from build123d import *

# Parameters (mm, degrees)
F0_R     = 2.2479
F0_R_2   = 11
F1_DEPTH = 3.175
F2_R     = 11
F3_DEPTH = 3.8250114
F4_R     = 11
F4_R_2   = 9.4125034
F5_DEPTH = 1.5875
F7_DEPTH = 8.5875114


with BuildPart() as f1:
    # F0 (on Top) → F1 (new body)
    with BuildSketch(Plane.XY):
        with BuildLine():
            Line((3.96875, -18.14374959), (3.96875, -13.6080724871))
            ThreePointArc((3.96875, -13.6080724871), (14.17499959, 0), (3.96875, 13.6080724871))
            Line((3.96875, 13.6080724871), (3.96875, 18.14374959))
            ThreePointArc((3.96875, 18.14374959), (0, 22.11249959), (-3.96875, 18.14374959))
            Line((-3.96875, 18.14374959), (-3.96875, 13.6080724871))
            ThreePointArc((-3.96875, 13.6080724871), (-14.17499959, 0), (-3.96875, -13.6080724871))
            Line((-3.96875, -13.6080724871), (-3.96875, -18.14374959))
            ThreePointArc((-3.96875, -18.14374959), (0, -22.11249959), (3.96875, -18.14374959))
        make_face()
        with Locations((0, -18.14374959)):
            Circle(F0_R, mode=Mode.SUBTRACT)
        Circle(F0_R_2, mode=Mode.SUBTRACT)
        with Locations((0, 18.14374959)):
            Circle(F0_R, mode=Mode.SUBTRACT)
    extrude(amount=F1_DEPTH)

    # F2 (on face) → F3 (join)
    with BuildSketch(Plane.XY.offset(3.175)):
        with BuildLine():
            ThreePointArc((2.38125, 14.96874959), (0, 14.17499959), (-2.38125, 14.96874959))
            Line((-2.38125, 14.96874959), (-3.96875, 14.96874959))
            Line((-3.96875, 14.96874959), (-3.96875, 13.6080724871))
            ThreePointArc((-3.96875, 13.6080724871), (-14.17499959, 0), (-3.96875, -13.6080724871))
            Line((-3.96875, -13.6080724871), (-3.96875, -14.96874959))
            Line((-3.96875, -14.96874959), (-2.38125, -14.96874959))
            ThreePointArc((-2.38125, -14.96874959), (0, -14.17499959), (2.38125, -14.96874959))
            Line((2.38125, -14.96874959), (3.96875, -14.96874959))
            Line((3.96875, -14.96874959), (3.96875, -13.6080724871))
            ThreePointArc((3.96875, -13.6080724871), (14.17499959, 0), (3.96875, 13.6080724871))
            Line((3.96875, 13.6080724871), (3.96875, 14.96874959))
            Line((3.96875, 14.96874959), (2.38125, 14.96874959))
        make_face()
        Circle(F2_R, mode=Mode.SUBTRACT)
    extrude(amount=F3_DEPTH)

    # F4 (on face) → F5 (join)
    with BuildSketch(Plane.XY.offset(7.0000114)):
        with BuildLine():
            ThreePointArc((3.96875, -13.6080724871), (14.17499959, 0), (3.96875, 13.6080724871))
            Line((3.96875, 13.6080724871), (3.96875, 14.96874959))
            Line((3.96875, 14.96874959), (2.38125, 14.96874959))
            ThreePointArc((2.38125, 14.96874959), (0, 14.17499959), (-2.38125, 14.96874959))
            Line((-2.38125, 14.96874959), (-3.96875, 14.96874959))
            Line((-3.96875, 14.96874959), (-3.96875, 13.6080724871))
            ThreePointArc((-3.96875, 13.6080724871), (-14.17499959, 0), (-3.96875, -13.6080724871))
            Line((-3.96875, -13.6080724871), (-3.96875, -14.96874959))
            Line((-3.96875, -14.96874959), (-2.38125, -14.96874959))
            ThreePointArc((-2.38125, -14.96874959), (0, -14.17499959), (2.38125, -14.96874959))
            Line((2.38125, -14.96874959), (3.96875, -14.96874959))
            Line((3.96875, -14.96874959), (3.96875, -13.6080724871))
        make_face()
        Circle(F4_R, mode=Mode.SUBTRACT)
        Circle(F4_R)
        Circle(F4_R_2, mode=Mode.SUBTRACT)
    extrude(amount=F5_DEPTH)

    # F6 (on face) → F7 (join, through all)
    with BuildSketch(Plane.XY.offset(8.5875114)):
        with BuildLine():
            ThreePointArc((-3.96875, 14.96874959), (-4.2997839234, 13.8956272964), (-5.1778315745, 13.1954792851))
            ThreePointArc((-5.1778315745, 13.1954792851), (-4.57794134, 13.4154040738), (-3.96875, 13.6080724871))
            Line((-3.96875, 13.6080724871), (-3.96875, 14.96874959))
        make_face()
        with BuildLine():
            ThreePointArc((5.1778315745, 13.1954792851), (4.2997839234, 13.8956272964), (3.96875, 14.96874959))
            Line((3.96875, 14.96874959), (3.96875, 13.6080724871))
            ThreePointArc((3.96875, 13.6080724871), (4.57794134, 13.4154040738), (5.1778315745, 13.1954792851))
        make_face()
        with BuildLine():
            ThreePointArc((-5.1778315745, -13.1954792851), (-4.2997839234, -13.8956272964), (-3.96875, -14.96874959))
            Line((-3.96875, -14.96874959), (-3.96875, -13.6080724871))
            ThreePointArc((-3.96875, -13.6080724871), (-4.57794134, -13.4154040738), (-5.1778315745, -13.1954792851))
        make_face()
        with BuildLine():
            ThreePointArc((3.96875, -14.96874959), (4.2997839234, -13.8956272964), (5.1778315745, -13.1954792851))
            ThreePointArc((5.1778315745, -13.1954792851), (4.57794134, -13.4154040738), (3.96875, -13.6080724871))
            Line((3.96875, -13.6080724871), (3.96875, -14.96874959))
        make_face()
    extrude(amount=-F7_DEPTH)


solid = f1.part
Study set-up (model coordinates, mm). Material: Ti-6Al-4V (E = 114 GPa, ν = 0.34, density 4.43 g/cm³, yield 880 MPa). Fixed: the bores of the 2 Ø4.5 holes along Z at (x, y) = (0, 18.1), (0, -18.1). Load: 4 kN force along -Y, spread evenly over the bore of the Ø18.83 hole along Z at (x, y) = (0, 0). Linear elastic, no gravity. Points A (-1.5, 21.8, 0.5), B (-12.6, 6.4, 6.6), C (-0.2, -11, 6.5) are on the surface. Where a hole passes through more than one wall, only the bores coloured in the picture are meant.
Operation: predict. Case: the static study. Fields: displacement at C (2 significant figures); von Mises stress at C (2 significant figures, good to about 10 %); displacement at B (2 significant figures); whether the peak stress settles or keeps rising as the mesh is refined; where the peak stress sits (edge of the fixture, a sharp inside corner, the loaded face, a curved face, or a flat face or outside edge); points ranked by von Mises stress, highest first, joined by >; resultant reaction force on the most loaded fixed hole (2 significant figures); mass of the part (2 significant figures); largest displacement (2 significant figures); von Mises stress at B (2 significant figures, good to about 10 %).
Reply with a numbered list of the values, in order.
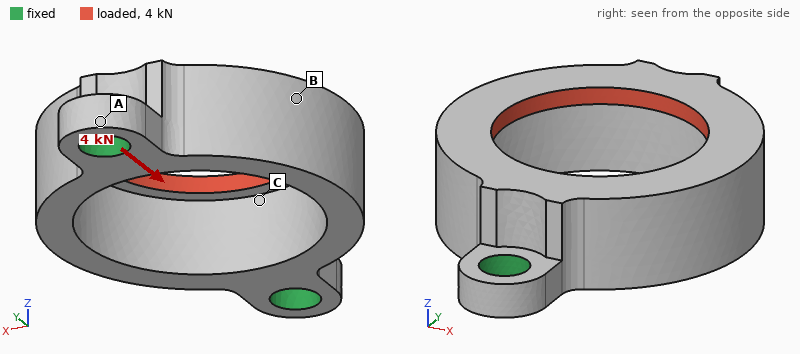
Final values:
1. 14 µm
2. 92 MPa
3. 20 µm
4. keeps rising
5. a sharp inside corner
6. C > B > A
7. 2.1 kN
8. 12 g
9. 26 µm
10. 57 MPa
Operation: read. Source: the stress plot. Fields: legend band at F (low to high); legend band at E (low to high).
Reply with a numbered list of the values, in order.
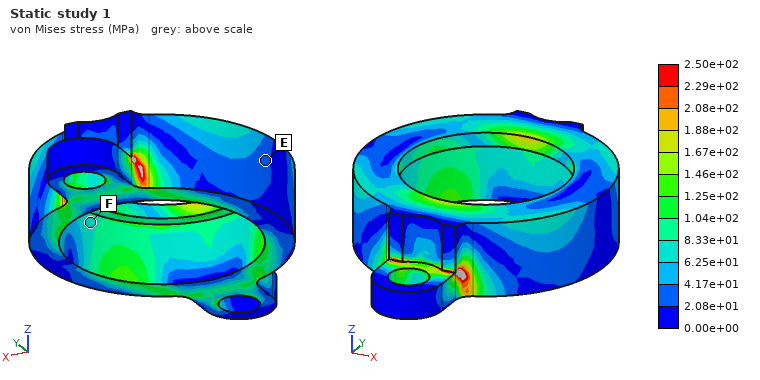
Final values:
1. 6.25e+01 to 8.33e+01 MPa
2. 2.08e+01 to 4.17e+01 MPa
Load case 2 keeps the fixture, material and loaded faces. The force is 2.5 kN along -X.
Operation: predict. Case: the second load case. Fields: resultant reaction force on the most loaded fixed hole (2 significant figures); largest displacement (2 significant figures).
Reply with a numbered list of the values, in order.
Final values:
1. 1.3 kN
2. 0.12 mm
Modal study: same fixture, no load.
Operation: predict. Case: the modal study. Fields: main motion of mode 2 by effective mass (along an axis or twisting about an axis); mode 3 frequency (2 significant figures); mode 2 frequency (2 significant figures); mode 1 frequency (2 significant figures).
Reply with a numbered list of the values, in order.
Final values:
1. along Z
2. 20 kHz
3. 13 kHz
4. 7600 Hz
